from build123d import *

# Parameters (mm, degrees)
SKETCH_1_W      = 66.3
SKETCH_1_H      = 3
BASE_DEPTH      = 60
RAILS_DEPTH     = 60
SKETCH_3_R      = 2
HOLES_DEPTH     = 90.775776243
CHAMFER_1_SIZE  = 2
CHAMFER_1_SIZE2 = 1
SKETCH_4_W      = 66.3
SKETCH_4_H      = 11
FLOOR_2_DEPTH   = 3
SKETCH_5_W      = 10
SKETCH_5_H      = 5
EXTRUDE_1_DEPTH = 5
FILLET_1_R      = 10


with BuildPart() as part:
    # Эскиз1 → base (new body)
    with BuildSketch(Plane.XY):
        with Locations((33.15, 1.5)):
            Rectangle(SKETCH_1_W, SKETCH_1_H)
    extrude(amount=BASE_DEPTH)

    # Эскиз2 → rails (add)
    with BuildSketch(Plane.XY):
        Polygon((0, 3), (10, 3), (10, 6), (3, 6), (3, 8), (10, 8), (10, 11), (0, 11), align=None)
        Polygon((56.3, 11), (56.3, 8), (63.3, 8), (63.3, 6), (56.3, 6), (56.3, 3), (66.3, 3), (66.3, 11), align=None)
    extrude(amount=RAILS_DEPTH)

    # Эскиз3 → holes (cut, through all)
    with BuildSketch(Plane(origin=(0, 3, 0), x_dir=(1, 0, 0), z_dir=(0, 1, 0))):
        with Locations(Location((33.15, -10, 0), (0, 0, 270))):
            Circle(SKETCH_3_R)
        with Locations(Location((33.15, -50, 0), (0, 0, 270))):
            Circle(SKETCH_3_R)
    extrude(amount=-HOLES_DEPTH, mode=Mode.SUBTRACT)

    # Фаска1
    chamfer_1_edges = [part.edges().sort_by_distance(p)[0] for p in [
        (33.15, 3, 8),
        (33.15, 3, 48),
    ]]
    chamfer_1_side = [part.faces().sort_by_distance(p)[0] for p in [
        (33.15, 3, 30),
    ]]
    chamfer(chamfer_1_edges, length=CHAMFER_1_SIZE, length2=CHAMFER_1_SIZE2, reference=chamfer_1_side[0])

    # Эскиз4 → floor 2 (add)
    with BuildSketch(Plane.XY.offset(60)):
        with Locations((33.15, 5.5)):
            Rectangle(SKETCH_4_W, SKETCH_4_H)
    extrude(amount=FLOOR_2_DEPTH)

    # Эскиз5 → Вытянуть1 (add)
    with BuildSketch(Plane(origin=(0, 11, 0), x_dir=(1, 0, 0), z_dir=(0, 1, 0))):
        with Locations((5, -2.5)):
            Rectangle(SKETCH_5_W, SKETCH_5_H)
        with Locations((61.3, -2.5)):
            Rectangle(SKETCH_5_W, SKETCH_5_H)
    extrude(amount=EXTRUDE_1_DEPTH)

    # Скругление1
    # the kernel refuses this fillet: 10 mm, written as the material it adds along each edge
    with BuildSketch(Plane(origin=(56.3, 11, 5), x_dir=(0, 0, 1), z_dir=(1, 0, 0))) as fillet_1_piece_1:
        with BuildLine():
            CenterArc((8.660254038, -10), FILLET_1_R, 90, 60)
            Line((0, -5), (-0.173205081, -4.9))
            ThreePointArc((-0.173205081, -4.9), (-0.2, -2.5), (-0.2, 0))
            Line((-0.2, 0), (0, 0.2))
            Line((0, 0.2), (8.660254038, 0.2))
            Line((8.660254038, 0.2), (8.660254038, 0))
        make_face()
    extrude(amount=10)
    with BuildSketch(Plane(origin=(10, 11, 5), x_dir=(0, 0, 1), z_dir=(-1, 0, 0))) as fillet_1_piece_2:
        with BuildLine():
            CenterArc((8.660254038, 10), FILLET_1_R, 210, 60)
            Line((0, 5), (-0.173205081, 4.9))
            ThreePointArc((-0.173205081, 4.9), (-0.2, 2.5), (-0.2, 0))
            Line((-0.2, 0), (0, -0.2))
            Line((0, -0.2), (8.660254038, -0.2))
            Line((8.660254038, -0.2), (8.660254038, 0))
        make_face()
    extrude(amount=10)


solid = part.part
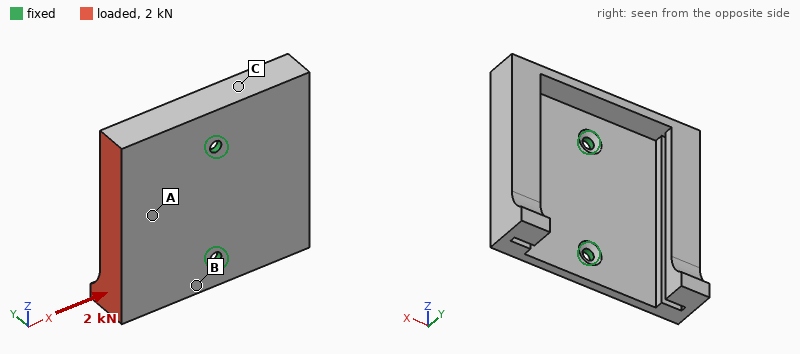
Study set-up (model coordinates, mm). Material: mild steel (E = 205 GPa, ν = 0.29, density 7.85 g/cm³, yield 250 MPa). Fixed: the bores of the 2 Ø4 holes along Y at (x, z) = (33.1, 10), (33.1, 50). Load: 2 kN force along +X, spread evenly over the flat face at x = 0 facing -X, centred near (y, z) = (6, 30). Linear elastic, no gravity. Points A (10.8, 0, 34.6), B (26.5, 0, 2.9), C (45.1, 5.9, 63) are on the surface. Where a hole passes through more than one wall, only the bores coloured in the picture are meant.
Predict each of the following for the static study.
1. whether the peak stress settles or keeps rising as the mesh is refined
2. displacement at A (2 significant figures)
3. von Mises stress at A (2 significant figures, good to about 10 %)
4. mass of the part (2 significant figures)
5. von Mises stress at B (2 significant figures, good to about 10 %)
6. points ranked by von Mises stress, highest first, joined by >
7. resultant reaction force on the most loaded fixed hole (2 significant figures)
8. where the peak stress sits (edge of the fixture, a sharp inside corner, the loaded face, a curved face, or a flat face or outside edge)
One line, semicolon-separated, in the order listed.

keeps rising; 0.069 mm; 33 MPa; 180 g; 56 MPa; B > A > C; 1.0 kN; edge of the fixture
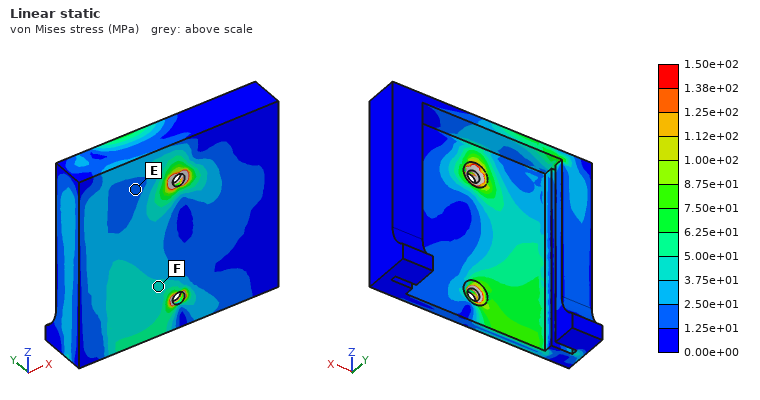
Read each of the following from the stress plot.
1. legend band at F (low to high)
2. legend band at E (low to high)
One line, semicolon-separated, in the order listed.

3.75e+01 to 5.00e+01 MPa; 1.25e+01 to 2.50e+01 MPa
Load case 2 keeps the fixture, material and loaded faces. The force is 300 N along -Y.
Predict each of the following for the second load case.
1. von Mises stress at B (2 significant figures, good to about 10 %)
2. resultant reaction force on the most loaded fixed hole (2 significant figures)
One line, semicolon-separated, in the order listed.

70 MPa; 160 N
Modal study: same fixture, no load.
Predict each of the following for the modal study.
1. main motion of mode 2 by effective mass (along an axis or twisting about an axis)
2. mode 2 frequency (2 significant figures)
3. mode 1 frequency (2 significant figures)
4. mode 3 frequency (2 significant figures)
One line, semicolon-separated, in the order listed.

along Y; 1800 Hz; 990 Hz; 2400 Hz
